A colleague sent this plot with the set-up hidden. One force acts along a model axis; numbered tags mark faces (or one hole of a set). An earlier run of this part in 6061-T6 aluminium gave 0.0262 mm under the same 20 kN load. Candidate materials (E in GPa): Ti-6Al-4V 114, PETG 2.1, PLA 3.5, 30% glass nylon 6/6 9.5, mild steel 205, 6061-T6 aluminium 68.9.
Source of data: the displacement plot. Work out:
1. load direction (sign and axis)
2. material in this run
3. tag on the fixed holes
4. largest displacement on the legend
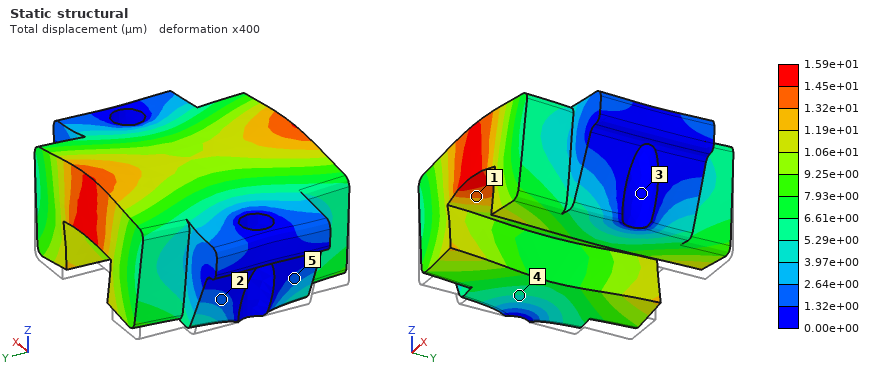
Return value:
+Z
Ti-6Al-4V
3
1.59e+01 µm
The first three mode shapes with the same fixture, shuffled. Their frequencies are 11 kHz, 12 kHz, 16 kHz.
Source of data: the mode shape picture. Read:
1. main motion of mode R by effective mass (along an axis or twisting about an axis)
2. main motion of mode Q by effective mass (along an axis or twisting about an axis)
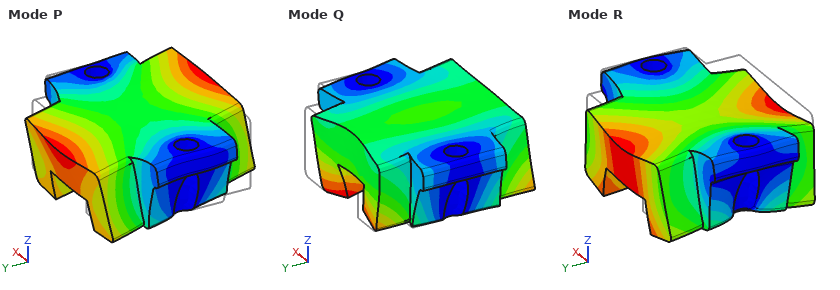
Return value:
along Z
along Y
